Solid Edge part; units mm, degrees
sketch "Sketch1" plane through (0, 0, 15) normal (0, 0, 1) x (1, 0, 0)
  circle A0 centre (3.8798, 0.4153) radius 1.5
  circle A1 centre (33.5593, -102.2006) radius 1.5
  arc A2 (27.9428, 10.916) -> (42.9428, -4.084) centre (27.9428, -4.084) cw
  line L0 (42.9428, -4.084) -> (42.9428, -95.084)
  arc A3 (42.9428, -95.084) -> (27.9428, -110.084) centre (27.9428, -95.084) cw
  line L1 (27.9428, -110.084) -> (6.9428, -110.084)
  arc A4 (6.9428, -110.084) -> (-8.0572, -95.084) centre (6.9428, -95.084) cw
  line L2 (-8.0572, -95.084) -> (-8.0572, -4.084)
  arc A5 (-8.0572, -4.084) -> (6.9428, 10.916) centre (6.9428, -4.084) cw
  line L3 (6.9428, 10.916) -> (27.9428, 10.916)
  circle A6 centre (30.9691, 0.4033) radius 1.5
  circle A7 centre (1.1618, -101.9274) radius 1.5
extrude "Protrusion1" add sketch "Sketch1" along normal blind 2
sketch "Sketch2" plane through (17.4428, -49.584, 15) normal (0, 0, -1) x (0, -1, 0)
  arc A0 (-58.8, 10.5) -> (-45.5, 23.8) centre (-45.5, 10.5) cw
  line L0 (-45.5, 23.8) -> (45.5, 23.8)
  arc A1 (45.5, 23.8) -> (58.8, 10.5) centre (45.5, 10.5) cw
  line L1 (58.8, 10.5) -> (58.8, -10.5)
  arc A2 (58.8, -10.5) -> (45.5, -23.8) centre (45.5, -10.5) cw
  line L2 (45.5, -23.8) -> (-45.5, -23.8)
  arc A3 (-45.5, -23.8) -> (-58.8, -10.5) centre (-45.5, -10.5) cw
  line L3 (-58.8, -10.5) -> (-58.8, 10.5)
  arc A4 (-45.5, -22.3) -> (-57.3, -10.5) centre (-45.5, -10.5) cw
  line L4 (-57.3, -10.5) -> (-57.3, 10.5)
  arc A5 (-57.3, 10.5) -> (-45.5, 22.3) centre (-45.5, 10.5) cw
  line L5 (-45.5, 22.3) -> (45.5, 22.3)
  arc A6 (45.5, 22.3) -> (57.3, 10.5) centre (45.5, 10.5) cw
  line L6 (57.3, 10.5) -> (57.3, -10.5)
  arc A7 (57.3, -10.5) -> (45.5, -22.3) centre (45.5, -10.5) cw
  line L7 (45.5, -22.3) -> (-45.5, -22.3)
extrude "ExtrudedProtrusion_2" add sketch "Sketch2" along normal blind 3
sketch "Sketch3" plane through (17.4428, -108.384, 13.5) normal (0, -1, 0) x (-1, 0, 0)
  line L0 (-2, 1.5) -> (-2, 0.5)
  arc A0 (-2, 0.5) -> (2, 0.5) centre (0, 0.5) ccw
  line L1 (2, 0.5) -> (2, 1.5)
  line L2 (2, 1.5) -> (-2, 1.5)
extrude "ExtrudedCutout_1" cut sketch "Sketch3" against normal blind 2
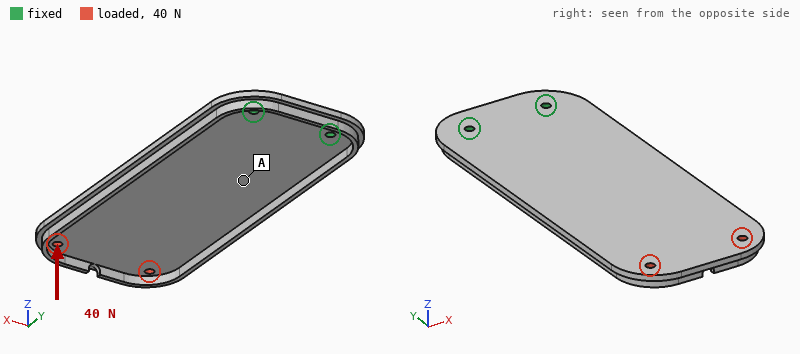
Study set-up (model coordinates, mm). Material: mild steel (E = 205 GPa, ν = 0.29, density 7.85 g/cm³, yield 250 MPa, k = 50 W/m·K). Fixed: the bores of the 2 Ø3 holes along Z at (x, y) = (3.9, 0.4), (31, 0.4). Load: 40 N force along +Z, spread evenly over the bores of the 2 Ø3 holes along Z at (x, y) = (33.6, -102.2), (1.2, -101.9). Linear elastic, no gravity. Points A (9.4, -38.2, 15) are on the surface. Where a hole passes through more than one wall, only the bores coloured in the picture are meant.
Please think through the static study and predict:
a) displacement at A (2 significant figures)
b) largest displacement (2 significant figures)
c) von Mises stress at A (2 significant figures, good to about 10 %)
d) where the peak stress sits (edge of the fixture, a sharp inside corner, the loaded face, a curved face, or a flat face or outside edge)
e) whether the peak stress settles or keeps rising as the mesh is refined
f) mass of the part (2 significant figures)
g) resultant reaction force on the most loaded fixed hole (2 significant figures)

0.21 mm
1.0 mm
21 MPa
edge of the fixture
keeps rising
100 g
63 N
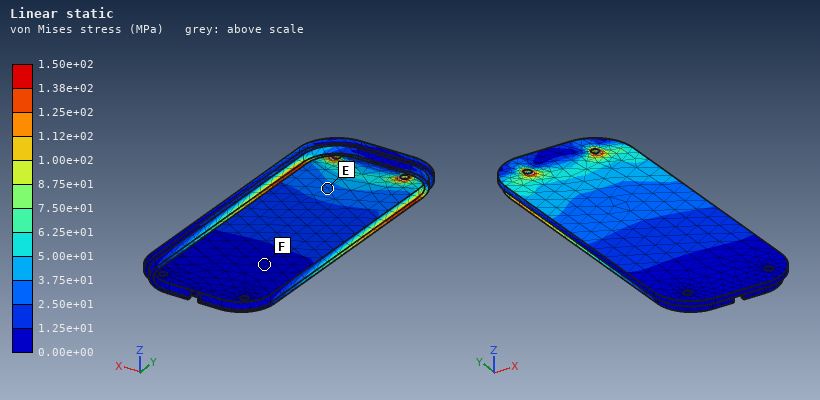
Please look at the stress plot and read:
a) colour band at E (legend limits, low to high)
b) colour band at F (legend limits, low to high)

2.50e+01 to 3.75e+01 MPa
0.00e+00 to 1.25e+01 MPa
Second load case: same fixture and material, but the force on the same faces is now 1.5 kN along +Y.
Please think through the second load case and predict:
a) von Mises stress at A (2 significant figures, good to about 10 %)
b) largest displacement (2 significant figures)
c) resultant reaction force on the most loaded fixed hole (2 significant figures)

11 MPa
85 µm
760 N
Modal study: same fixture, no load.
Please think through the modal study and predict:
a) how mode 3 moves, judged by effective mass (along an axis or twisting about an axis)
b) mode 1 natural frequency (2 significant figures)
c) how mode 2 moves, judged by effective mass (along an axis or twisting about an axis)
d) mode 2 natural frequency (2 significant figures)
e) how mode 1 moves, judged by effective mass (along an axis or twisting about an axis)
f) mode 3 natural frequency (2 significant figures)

along Z
190 Hz
twisting about Y
670 Hz
along Z
1200 Hz
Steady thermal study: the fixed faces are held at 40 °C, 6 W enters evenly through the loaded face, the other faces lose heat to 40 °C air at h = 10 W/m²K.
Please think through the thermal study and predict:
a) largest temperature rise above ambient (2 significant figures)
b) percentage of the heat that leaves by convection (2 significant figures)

68 K
64 %
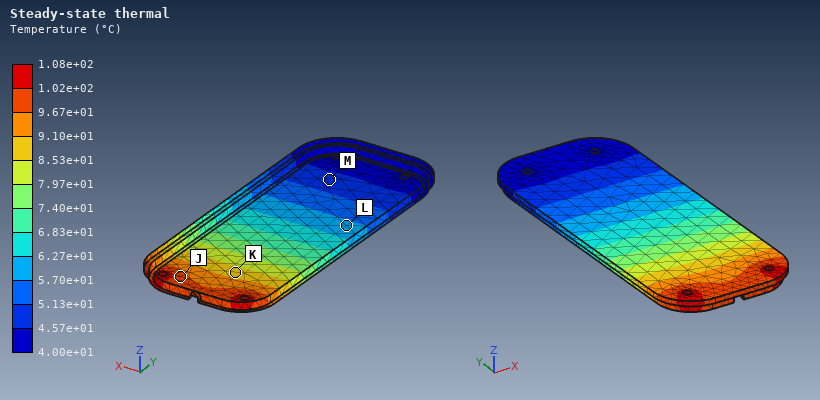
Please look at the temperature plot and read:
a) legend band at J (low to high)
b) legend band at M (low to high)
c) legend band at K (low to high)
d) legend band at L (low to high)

9.67e+01 to 1.02e+02 °C
4.57e+01 to 5.13e+01 °C
8.53e+01 to 9.10e+01 °C
5.70e+01 to 6.27e+01 °C
